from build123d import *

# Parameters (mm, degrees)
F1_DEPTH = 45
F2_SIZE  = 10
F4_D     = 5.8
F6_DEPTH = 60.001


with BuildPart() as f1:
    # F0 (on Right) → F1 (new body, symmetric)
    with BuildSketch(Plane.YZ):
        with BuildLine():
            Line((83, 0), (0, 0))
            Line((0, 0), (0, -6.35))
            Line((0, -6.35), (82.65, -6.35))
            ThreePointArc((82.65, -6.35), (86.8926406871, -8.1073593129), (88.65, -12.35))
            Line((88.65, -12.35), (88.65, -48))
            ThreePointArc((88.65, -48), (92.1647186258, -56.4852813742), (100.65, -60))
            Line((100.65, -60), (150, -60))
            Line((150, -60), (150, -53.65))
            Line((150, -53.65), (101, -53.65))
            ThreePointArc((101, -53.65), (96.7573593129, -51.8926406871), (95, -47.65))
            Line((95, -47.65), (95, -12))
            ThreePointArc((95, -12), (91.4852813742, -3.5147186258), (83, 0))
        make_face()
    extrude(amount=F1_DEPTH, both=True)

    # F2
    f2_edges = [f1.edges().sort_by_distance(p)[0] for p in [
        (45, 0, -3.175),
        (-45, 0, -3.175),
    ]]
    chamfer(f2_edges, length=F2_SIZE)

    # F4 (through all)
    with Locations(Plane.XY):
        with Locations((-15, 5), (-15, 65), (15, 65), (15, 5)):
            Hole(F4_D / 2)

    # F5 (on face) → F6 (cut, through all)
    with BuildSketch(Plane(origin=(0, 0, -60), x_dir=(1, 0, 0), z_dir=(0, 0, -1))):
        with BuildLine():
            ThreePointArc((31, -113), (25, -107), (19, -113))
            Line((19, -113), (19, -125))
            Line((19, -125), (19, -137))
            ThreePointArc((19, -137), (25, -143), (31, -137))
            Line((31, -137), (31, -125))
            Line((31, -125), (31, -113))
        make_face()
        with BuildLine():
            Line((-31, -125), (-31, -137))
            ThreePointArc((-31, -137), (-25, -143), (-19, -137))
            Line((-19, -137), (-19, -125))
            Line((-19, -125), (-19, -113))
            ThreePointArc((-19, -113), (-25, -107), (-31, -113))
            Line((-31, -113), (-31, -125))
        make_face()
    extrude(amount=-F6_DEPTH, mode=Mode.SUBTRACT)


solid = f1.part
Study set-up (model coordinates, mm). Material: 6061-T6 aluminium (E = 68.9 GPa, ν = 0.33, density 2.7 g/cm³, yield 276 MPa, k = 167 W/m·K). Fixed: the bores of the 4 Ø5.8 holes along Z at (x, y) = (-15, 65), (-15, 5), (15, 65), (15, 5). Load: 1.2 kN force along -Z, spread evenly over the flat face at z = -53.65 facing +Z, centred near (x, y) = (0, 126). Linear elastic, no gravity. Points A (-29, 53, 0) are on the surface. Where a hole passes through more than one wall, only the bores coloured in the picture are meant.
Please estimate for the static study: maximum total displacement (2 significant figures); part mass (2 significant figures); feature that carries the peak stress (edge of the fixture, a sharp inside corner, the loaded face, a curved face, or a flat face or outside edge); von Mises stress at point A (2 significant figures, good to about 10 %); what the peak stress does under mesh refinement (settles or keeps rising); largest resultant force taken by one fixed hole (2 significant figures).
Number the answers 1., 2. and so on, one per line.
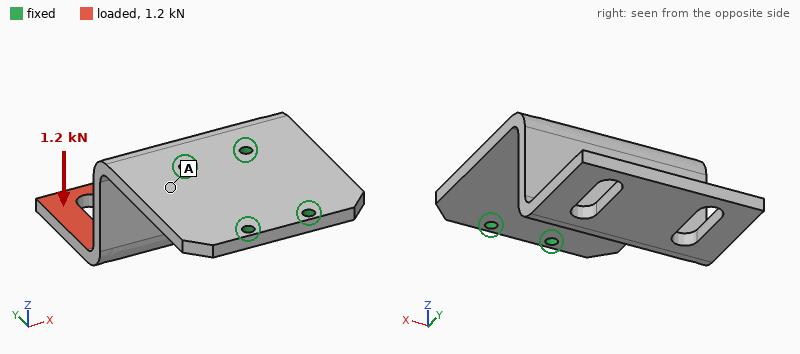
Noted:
1. 2.2 mm
2. 290 g
3. edge of the fixture
4. 21 MPa
5. keeps rising
6. 770 N
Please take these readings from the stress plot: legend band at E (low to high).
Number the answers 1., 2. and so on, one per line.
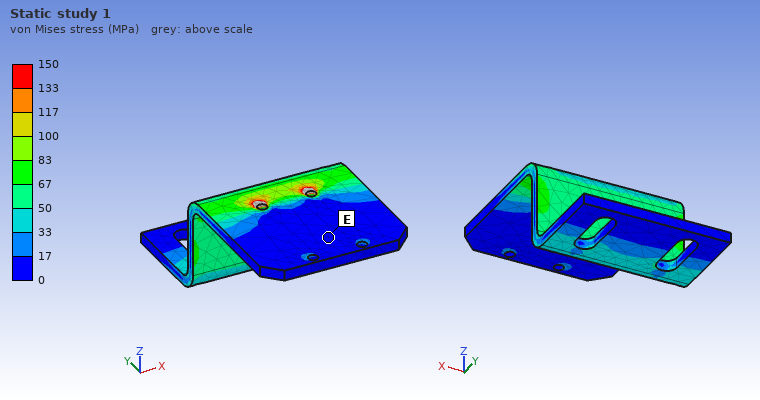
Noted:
1. 0 to 17 MPa
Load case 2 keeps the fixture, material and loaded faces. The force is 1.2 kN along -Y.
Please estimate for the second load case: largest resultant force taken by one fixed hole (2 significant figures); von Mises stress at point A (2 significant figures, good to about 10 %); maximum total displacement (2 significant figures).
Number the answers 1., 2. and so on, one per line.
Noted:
1. 560 N
2. 18 MPa
3. 1.7 mm
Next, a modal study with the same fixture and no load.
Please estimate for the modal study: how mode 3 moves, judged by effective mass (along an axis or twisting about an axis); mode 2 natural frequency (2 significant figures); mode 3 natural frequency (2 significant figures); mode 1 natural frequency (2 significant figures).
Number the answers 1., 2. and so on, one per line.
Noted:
1. along X
2. 1000 Hz
3. 1200 Hz
4. 420 Hz
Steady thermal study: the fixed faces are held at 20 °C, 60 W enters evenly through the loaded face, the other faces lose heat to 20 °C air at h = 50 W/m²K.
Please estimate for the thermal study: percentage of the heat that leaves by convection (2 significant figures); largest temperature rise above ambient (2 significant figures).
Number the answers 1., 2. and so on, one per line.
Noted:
1. 46 %
2. 50 K
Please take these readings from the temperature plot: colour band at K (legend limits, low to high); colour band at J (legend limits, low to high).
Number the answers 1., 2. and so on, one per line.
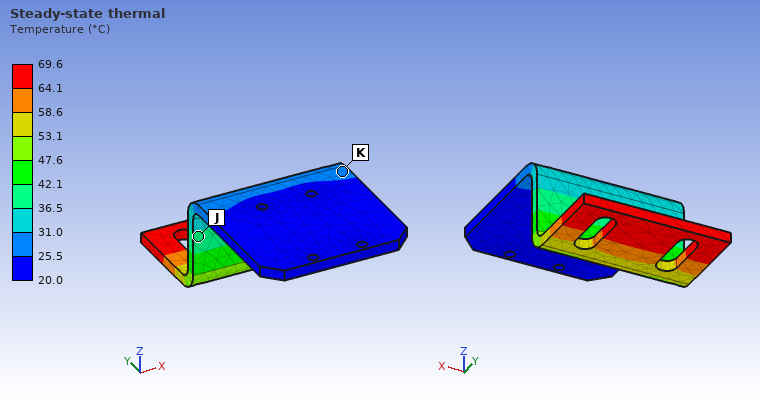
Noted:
1. 25.5 to 31.0 °C
2. 36.5 to 42.1 °C
